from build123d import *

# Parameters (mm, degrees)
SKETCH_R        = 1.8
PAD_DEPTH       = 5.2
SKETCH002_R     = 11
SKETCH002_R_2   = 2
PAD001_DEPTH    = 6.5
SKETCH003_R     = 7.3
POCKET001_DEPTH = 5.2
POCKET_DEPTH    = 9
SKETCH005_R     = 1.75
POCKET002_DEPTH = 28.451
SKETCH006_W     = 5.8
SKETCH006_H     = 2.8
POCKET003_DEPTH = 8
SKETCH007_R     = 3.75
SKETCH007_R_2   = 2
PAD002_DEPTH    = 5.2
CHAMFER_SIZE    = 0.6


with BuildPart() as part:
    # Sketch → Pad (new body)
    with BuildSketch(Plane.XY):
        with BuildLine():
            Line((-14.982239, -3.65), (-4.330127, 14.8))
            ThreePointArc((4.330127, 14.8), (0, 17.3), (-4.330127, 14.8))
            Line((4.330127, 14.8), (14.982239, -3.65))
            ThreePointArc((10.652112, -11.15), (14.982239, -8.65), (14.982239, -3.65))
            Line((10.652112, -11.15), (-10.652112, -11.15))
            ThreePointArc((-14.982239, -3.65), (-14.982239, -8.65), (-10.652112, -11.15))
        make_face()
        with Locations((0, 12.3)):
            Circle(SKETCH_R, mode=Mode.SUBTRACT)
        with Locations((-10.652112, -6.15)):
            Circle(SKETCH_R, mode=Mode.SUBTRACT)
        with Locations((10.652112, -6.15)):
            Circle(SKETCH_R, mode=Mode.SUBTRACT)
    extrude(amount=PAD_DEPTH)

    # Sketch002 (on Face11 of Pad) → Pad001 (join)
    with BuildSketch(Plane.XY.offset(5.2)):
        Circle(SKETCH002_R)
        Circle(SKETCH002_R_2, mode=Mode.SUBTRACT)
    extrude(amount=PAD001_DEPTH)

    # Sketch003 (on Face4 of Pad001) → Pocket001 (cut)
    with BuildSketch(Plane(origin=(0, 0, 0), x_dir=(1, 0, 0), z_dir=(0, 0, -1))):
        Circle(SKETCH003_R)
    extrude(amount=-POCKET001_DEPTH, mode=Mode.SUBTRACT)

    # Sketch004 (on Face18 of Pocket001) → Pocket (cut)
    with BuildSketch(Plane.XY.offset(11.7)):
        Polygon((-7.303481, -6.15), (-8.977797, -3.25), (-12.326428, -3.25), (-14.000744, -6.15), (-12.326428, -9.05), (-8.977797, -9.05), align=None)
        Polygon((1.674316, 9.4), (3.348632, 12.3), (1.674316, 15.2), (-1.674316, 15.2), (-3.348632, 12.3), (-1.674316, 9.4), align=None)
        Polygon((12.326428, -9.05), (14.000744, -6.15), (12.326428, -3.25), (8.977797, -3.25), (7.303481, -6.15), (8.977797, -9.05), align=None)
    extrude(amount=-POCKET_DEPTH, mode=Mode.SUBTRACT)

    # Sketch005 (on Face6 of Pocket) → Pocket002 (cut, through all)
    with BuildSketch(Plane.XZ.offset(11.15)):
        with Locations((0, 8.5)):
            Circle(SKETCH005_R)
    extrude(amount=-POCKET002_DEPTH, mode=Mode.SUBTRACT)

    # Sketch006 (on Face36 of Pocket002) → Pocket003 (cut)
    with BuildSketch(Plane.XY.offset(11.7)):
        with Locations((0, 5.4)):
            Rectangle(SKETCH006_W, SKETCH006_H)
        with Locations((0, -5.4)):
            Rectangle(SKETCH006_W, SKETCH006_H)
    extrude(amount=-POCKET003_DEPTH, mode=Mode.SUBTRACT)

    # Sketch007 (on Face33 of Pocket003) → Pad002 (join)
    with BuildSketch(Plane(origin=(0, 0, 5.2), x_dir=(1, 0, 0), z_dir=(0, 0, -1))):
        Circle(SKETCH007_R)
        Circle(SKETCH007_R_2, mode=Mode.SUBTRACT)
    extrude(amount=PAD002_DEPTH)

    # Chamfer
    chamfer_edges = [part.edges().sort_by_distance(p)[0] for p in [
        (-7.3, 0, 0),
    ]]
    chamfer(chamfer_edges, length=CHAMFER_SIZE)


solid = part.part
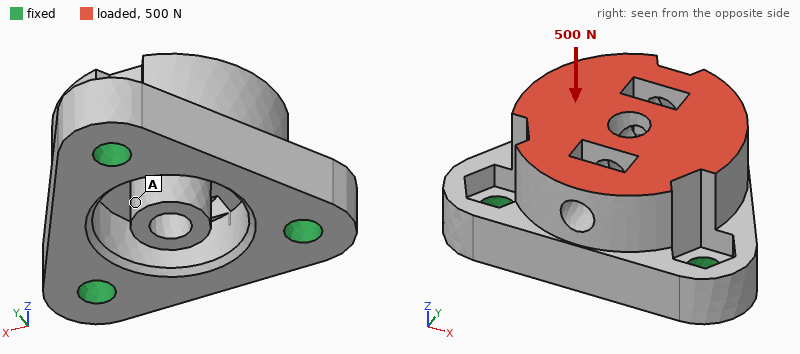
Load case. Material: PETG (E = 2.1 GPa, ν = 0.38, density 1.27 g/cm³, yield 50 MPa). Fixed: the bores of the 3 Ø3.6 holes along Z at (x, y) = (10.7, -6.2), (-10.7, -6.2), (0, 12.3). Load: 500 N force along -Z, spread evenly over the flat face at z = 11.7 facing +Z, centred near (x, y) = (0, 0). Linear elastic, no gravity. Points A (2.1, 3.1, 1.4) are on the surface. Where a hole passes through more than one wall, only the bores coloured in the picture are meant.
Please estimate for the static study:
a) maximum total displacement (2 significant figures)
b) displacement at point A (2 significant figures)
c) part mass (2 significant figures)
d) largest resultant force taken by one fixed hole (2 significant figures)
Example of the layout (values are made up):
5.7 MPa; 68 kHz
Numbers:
54 µm; 46 µm; 5.1 g; 180 N
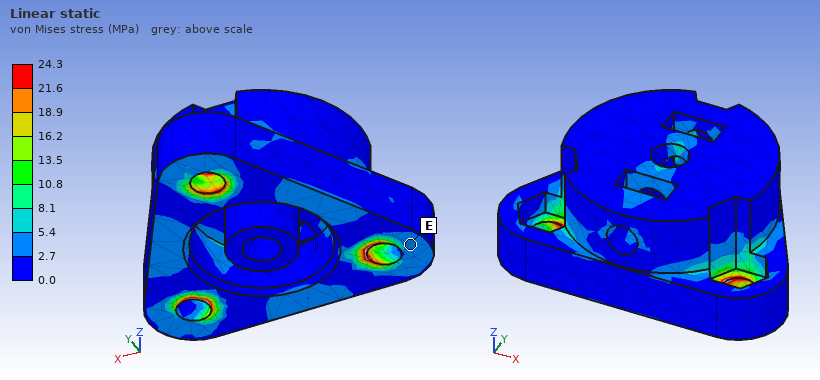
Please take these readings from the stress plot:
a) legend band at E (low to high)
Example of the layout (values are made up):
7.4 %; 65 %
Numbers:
2.7 to 5.4 MPa
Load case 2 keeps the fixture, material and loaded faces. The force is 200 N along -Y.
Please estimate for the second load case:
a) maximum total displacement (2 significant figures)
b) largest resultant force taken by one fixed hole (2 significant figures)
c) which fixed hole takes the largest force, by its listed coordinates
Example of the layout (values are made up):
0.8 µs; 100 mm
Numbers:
60 µm; 140 N; (0, 12.3)
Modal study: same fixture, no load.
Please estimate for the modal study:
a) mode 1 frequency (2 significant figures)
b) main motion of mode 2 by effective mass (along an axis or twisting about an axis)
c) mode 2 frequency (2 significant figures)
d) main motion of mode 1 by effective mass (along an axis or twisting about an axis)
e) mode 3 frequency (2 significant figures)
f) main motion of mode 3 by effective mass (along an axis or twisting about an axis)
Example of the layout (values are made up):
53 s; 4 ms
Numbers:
7400 Hz; along Y; 7800 Hz; along X; 8900 Hz; along Z
